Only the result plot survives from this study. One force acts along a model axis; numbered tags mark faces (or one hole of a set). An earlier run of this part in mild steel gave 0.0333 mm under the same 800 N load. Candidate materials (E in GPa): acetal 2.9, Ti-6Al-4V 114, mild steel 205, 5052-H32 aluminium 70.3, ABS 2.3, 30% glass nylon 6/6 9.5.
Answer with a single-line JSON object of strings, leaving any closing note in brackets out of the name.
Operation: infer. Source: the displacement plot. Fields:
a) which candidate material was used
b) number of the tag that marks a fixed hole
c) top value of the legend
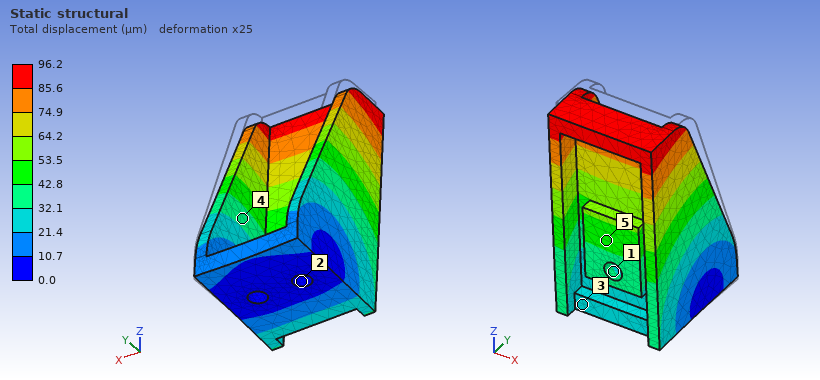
{"which candidate material was used": "5052-H32 aluminium", "number of the tag that marks a fixed hole": "2", "top value of the legend": "96.2 µm"}
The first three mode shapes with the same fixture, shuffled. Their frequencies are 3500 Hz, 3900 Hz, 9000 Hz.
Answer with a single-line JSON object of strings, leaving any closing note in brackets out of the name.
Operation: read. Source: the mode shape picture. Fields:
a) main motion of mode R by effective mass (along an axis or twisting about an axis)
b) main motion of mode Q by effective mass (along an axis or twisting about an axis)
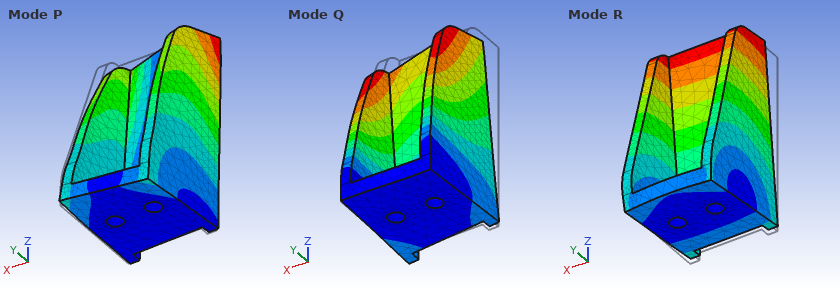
{"main motion of mode R by effective mass": "along Y", "main motion of mode Q by effective mass": "along X"}
